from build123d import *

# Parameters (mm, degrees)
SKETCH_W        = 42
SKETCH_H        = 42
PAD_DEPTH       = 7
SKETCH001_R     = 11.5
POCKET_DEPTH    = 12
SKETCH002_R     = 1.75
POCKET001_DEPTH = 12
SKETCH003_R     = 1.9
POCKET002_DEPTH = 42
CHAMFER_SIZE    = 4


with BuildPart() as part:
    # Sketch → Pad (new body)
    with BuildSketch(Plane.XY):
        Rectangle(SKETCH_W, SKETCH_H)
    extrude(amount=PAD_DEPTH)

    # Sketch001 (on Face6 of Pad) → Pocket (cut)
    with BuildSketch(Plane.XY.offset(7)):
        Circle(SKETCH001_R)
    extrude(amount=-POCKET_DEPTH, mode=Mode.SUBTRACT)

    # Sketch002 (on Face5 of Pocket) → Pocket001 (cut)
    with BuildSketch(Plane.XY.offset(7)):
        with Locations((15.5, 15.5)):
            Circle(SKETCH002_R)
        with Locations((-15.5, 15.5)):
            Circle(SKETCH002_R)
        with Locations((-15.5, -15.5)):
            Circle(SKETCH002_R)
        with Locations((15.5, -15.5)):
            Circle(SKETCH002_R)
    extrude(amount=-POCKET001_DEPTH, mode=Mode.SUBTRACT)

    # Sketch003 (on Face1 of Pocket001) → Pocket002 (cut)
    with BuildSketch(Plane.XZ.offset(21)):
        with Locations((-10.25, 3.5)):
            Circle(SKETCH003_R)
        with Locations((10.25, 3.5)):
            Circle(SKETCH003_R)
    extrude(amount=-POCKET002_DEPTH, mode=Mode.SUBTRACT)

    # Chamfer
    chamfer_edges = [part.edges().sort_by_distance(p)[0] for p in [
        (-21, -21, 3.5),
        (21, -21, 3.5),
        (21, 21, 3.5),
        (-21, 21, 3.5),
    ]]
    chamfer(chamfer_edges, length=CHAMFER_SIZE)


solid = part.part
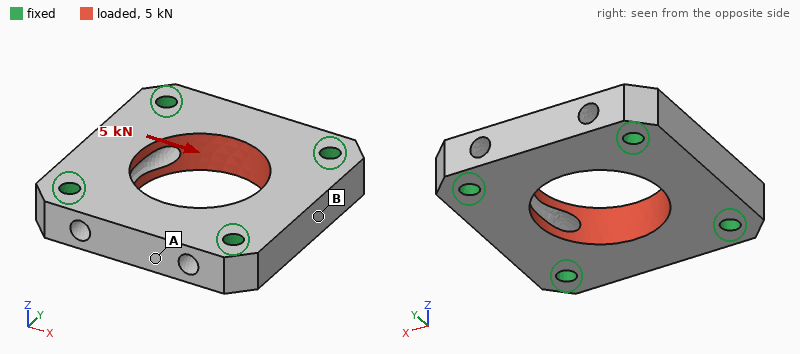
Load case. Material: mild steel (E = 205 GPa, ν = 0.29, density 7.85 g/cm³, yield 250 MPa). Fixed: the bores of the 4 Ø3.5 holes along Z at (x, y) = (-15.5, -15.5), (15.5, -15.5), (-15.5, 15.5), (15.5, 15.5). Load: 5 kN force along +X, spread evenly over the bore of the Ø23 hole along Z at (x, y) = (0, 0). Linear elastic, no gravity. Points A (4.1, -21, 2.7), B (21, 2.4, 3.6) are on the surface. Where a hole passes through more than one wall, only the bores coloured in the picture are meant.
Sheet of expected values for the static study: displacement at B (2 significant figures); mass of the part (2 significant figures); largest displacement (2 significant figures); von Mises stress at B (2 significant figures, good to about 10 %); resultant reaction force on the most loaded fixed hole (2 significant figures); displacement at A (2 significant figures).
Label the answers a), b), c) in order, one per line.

a) 1.7 µm
b) 64 g
c) 2.7 µm
d) 17 MPa
e) 1.3 kN
f) 0.73 µm
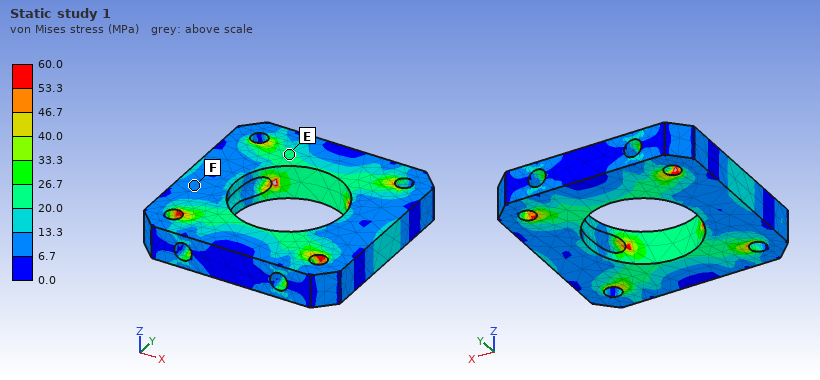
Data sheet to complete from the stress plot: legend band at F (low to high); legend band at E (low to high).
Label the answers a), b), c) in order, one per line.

a) 6.7 to 13.3 MPa
b) 20.0 to 26.7 MPa
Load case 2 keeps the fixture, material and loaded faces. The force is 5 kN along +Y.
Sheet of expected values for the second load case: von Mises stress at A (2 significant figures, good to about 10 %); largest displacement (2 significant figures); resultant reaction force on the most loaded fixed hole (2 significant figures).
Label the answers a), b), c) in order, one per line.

a) 22 MPa
b) 3.4 µm
c) 1.3 kN
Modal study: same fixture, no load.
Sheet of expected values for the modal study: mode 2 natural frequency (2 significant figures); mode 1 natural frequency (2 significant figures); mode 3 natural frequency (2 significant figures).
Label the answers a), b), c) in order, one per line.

a) 25 kHz
b) 25 kHz
c) 28 kHz
